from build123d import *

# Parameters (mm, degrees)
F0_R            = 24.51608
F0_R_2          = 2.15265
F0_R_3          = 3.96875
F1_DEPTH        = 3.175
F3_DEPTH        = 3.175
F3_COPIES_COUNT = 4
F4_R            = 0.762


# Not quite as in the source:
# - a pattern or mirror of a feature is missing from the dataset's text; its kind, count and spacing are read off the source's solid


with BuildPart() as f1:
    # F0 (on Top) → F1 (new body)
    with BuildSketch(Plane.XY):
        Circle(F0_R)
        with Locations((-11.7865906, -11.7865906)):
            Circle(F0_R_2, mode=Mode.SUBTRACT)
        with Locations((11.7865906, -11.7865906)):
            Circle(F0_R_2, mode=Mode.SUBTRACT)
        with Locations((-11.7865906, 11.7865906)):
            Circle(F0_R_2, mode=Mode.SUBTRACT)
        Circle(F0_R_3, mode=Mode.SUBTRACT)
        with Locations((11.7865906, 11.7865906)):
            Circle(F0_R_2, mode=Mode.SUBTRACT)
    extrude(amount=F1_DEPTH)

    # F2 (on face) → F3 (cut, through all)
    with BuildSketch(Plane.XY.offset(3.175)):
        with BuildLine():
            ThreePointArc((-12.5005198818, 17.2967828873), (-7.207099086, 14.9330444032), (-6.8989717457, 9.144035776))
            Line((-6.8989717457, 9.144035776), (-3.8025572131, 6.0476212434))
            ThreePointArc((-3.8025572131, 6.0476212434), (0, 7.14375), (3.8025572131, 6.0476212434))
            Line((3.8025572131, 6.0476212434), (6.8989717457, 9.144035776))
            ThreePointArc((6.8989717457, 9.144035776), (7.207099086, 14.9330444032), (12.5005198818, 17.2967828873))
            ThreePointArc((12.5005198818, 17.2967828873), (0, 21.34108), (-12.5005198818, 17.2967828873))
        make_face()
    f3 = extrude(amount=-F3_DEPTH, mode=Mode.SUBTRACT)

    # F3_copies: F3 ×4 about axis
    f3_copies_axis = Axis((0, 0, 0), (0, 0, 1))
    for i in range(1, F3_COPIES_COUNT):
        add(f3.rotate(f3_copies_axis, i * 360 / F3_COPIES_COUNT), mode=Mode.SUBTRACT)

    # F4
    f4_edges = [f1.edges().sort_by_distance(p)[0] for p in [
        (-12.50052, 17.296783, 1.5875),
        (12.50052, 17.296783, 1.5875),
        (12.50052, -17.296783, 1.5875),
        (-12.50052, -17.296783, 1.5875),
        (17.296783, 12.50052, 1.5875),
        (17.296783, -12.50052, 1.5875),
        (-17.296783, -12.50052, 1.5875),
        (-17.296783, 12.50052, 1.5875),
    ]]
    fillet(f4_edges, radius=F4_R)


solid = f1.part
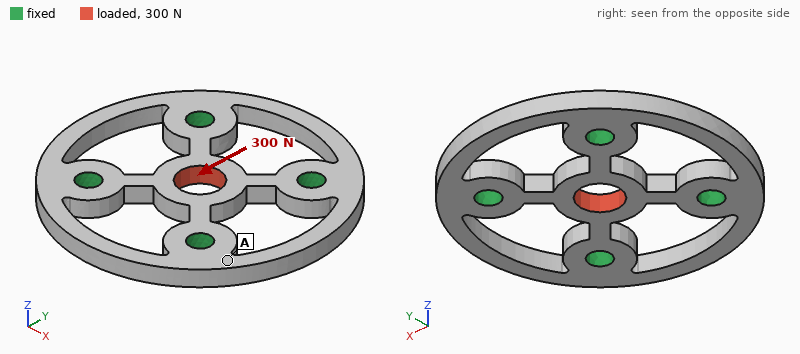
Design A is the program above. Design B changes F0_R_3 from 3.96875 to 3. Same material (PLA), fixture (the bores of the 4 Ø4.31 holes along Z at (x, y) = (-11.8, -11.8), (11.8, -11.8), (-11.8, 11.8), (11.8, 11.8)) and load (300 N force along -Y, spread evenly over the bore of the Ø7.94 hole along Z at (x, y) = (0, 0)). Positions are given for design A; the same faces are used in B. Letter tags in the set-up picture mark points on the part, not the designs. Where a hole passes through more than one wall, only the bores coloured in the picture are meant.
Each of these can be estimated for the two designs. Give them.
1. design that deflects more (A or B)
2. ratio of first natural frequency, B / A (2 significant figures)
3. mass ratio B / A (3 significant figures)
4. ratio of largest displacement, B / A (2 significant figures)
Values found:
A
1.00
1.02
0.84
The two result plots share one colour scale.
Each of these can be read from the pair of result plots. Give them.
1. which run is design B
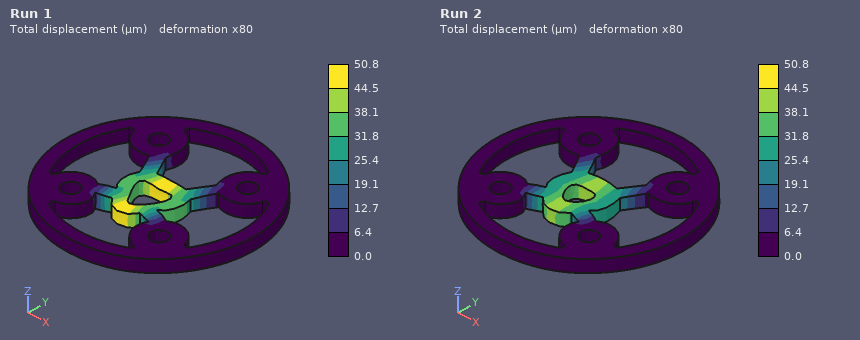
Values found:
Run 2
